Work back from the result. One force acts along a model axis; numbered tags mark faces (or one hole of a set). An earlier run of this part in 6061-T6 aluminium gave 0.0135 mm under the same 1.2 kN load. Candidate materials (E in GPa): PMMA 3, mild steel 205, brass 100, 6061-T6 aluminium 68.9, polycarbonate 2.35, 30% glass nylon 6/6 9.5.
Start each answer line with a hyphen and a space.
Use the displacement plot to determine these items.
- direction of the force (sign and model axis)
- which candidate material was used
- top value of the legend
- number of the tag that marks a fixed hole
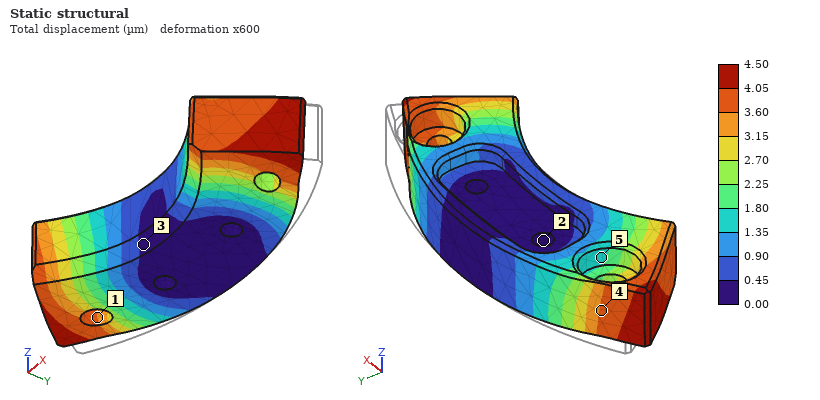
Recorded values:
- -Y
- mild steel
- 4.50 µm
- 2
